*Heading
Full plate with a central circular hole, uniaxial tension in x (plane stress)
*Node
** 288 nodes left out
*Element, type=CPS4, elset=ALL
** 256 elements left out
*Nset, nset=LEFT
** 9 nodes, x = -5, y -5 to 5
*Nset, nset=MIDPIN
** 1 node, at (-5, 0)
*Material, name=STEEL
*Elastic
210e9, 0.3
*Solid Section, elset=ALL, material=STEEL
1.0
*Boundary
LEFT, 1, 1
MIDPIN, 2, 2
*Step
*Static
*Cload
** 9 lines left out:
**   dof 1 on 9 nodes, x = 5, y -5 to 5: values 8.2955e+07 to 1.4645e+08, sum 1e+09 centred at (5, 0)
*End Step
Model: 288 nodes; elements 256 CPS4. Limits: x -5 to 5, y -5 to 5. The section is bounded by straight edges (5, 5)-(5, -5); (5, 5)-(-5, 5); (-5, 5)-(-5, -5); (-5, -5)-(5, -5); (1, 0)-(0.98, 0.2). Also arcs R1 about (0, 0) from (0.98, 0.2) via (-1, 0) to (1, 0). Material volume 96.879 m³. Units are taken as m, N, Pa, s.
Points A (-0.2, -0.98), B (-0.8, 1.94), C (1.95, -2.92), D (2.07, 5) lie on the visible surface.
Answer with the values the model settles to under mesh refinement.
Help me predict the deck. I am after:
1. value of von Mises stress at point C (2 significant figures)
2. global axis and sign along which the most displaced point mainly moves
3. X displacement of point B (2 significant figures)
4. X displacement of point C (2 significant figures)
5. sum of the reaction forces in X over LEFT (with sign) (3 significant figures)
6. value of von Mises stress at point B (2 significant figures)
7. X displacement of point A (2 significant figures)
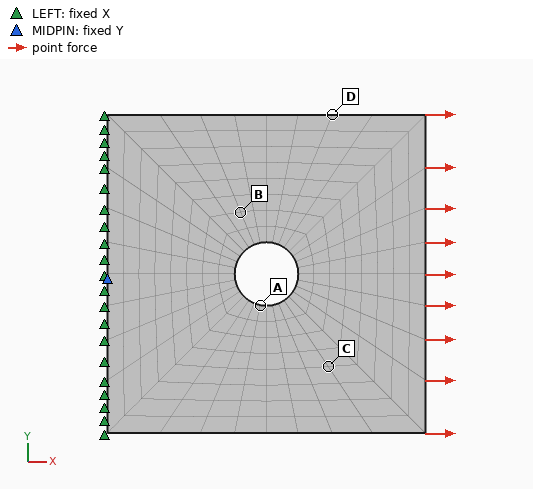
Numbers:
1.1e+08 Pa
+X
0.0022 m
0.0036 m
-1.00e+09 N
1.3e+08 Pa
0.0024 m
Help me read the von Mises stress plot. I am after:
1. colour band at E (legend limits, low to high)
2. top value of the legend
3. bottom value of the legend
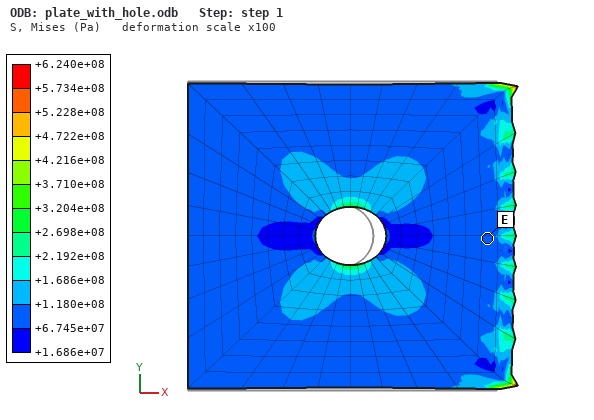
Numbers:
+6.745e+07 to +1.180e+08 Pa
+6.240e+08 Pa
+1.686e+07 Pa
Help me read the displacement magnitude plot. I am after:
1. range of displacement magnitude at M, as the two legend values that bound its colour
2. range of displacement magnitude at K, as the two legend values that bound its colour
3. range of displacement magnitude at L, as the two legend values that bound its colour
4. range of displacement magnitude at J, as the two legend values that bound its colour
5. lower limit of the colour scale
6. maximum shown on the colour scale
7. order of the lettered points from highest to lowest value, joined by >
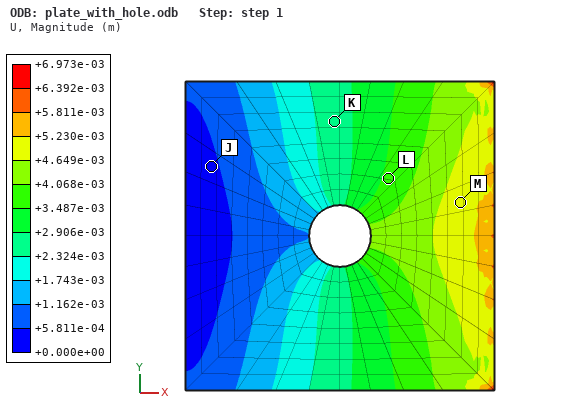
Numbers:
+4.649e-03 to +5.230e-03 m
+2.324e-03 to +2.906e-03 m
+3.487e-03 to +4.068e-03 m
+0.000e+00 to +5.811e-04 m
+0.000e+00 m
+6.973e-03 m
M > L > K > J
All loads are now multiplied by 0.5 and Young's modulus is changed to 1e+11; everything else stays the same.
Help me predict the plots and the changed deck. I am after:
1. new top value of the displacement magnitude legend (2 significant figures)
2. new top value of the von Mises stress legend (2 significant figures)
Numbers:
0.0073 m
3.1e+08 Pa
